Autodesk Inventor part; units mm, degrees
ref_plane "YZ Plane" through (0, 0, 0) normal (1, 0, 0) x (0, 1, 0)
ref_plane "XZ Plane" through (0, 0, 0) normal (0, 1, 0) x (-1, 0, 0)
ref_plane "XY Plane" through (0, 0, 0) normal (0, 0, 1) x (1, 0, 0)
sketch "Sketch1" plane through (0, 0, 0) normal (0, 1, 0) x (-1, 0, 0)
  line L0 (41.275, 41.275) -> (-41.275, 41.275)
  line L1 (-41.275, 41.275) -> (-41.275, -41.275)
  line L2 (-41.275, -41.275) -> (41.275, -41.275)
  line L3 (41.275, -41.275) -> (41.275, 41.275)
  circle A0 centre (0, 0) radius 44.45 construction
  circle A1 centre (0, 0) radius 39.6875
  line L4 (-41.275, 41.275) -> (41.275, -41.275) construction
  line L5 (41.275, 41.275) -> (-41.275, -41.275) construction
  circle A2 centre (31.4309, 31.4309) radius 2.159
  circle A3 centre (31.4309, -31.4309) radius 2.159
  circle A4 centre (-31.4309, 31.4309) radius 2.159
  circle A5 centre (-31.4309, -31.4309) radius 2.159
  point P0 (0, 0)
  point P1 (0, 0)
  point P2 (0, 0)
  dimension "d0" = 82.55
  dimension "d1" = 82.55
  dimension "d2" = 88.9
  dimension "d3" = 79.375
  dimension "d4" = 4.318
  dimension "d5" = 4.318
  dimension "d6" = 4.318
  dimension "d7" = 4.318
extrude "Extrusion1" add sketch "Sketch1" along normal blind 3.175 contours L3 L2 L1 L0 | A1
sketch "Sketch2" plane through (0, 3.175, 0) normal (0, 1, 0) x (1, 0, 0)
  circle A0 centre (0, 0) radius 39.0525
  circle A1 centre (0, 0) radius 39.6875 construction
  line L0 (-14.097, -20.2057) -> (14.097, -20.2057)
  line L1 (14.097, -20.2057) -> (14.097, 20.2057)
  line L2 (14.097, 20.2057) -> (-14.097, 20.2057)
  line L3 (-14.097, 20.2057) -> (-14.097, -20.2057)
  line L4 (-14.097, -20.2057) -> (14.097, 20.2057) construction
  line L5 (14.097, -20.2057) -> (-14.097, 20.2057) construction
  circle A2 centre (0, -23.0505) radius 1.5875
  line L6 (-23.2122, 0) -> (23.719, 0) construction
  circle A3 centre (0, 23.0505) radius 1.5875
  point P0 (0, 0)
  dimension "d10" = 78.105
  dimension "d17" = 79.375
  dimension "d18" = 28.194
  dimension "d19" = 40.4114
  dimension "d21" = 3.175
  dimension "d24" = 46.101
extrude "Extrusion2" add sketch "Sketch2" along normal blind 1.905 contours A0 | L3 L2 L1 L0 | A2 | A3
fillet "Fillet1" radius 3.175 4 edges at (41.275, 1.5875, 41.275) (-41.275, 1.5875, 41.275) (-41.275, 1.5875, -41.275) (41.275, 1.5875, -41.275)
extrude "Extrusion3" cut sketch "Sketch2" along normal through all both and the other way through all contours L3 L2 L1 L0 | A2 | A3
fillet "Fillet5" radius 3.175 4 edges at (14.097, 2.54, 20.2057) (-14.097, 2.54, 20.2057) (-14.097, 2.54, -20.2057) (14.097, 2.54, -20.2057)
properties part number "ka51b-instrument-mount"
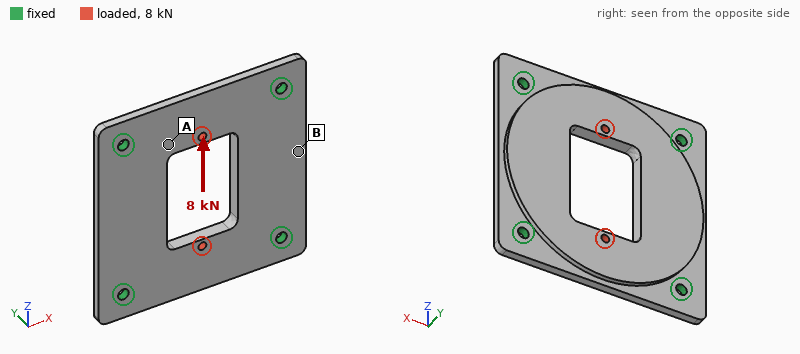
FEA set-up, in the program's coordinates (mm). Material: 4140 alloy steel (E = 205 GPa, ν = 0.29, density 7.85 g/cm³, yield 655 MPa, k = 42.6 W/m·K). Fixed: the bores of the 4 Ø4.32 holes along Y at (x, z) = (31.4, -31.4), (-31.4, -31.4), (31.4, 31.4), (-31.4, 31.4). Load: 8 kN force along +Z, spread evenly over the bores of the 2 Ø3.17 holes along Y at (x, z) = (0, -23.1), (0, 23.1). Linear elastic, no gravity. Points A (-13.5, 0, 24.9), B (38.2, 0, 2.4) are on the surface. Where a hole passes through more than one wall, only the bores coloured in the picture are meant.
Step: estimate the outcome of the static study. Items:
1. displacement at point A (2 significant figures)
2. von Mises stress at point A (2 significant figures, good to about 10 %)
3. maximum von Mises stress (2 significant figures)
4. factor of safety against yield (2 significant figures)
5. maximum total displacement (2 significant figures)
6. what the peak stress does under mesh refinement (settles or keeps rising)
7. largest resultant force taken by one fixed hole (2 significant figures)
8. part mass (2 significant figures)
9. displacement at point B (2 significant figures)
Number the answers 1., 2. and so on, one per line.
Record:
1. 6.7 µm
2. 43 MPa
3. 260 MPa
4. 2.5
5. 17 µm
6. settles
7. 2.1 kN
8. 190 g
9. 2.9 µm
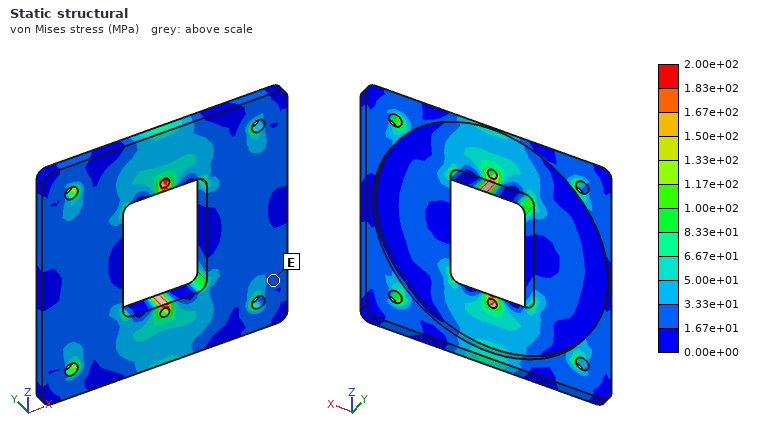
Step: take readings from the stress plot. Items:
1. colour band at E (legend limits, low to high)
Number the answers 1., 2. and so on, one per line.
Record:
1. 1.67e+01 to 3.33e+01 MPa
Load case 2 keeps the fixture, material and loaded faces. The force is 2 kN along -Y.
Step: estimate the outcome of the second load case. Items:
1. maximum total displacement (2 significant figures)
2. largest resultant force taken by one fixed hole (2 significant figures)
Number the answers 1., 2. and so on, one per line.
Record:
1. 70 µm
2. 1.1 kN
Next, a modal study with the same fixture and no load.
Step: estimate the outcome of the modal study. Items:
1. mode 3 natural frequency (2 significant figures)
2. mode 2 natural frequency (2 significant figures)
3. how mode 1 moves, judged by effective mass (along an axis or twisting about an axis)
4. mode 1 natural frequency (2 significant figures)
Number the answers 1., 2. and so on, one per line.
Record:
1. 5300 Hz
2. 5300 Hz
3. along Y
4. 4000 Hz
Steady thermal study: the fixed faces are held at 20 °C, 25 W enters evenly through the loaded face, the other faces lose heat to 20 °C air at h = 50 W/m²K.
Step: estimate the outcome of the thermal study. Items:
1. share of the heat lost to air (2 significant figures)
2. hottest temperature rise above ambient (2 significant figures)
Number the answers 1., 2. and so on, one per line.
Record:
1. 37 %
2. 59 K
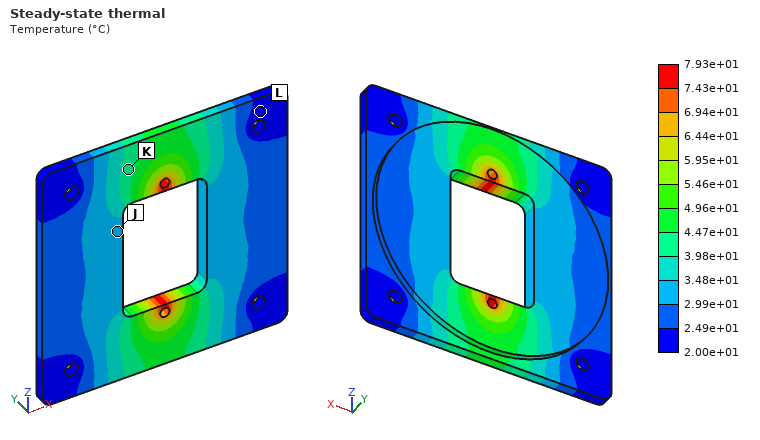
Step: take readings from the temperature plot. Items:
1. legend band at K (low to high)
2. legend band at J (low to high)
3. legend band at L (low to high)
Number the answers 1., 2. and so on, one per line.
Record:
1. 3.98e+01 to 4.47e+01 °C
2. 2.99e+01 to 3.48e+01 °C
3. 2.00e+01 to 2.49e+01 °C
